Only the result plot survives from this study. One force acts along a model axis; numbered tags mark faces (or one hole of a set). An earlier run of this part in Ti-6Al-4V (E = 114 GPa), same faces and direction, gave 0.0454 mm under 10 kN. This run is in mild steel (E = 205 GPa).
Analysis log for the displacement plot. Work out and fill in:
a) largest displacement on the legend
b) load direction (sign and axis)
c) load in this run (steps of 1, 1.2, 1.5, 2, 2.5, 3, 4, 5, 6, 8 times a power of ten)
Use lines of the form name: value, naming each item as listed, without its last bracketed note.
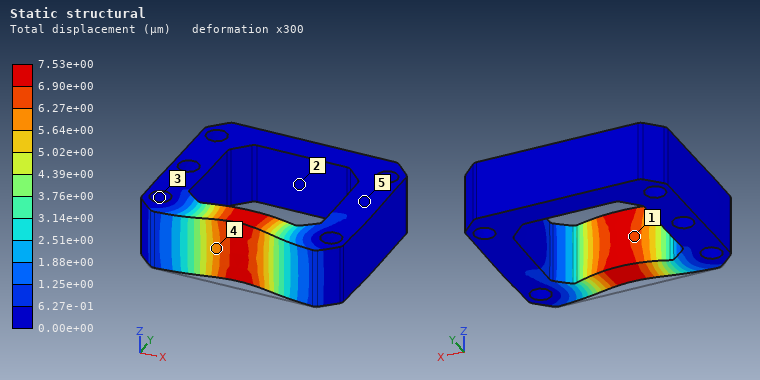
largest displacement on the legend: 7.53e+00 µm
load direction: +Y
load in this run: 3 kN
